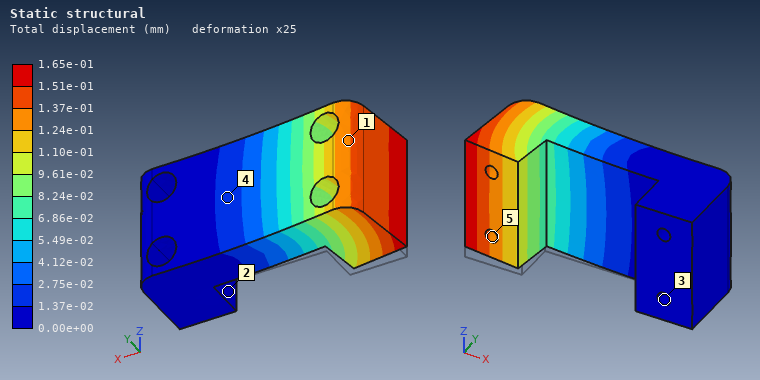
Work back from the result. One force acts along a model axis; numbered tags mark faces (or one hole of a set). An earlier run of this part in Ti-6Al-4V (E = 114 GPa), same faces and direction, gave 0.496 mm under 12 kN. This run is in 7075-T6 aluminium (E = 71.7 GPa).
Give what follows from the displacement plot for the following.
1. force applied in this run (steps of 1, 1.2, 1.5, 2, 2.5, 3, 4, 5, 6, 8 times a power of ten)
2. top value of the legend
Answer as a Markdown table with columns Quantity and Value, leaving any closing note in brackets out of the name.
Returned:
| Quantity | Value |
|---|---|
| force applied in this run | 2.5 kN |
| top value of the legend | 1.65e-01 mm |
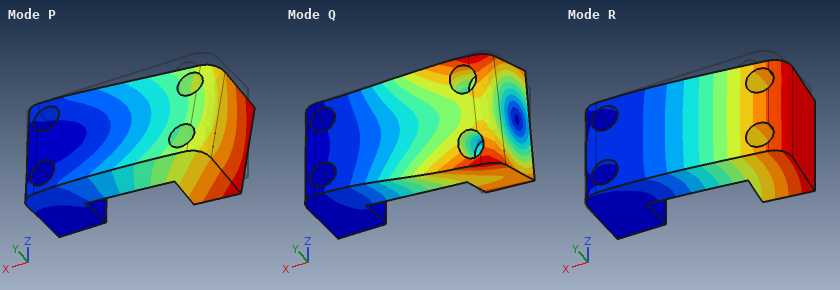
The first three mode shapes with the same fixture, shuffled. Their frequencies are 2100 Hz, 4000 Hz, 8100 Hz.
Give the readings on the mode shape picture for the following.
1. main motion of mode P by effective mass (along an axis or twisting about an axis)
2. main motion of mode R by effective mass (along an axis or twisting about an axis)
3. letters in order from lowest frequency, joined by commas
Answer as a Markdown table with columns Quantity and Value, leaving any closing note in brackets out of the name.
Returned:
| Quantity | Value |
|---|---|
| main motion of mode P by effective mass | along Z |
| main motion of mode R by effective mass | along Y |
| letters in order from lowest frequency, joined by commas | R, P, Q |
